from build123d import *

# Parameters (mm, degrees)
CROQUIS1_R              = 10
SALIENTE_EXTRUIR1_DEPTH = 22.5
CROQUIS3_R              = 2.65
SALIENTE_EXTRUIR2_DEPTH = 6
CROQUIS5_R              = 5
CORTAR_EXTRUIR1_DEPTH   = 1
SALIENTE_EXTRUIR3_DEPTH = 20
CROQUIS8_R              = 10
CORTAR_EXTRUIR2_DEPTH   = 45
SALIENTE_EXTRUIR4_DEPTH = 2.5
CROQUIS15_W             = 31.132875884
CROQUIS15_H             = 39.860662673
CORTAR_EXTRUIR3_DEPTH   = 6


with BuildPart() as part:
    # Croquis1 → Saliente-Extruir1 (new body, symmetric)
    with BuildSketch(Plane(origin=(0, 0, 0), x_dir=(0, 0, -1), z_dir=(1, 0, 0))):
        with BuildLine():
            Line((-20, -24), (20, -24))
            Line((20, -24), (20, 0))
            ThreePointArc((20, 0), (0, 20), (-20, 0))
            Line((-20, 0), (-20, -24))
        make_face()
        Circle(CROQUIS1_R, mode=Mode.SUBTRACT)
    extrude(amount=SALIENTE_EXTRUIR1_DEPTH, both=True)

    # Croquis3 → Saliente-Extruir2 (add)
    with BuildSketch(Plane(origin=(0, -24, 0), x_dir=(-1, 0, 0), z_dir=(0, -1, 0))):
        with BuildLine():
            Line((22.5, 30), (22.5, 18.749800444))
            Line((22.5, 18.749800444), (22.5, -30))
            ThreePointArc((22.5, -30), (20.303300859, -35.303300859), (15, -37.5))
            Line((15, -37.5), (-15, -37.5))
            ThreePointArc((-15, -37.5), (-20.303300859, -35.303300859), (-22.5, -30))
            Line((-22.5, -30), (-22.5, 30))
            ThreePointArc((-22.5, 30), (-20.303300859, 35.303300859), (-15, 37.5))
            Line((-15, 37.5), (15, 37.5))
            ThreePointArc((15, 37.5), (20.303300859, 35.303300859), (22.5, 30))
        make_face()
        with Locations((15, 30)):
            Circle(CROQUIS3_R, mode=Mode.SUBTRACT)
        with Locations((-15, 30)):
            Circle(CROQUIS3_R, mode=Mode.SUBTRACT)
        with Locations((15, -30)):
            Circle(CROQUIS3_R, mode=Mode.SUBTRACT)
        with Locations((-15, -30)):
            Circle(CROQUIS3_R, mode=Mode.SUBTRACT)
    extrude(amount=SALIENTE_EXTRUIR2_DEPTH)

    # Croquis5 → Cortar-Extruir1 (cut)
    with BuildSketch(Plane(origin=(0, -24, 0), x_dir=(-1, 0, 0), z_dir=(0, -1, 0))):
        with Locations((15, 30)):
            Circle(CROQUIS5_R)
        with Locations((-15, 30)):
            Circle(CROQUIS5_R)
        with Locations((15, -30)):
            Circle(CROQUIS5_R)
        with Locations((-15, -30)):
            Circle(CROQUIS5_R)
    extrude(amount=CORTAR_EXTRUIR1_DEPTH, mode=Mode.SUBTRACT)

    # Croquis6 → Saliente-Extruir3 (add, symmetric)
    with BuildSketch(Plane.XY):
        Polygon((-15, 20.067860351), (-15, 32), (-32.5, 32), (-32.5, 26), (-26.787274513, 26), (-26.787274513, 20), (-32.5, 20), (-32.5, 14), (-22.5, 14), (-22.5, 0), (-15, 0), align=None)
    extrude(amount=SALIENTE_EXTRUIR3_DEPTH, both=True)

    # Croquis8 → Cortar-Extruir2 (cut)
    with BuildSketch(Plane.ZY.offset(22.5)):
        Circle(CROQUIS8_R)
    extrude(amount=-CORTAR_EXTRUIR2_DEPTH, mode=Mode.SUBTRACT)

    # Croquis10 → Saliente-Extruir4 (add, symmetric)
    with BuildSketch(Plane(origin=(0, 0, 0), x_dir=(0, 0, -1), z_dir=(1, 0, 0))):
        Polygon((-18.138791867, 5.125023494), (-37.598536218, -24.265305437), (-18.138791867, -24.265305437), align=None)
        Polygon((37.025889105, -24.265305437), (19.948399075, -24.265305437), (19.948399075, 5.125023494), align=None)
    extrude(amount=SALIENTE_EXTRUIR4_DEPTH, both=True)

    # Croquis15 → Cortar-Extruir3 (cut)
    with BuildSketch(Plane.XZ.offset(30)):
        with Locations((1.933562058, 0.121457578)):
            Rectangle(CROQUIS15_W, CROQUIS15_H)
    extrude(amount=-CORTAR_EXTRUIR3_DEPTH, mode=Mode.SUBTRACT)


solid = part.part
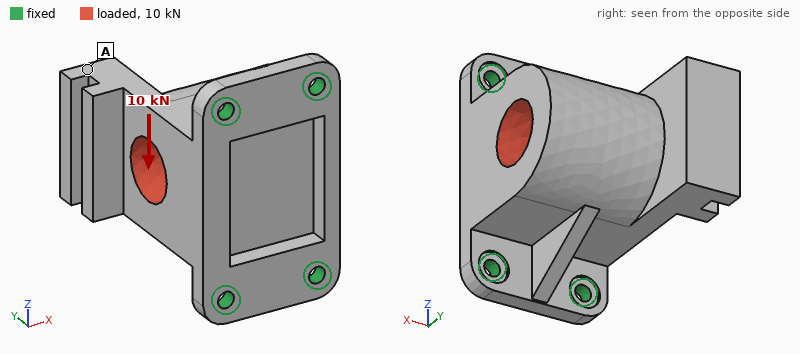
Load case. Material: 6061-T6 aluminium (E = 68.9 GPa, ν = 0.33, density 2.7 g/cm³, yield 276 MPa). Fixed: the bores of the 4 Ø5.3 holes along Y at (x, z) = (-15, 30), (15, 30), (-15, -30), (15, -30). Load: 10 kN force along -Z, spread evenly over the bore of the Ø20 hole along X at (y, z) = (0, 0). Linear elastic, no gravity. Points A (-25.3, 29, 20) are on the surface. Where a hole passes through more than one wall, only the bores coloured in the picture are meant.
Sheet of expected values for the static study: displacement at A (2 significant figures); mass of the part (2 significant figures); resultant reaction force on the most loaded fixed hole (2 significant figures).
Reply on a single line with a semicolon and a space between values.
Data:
77 µm; 220 g; 3.9 kN
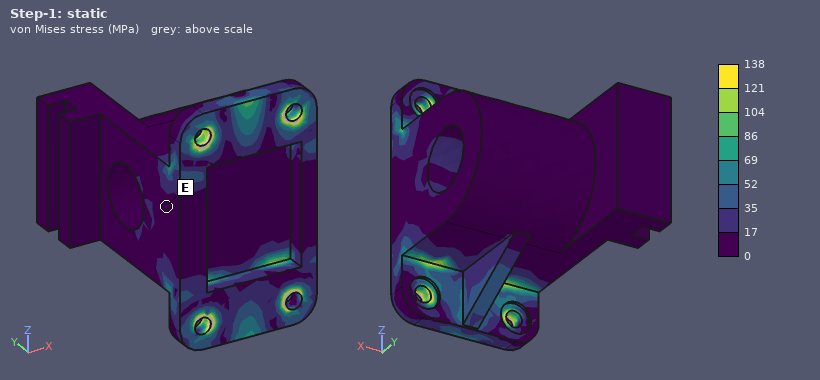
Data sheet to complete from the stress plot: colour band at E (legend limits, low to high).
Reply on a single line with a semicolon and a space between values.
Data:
0 to 17 MPa
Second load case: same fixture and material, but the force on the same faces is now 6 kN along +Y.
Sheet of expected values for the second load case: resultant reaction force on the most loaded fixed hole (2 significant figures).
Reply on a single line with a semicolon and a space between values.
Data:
1.9 kN
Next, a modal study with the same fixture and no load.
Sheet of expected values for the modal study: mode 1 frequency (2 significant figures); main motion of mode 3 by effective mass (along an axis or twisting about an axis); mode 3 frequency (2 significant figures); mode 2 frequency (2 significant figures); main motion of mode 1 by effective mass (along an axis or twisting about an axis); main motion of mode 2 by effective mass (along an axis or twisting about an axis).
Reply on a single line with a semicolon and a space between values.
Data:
2500 Hz; along Y; 6300 Hz; 4700 Hz; along X; along Z
